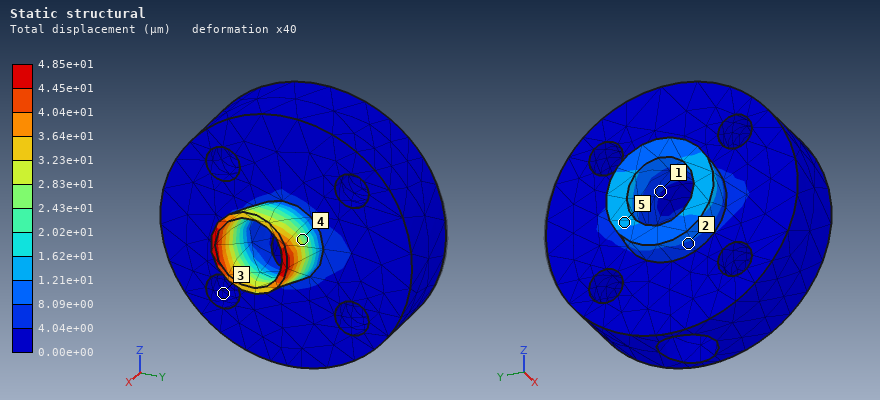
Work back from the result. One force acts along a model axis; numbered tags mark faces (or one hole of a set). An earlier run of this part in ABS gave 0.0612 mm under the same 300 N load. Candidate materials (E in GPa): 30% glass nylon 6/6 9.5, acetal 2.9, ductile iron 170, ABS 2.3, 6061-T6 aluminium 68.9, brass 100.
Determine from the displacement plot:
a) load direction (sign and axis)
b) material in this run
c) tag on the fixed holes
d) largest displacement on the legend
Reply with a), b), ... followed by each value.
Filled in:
a) -Y
b) acetal
c) 3
d) 4.85e+01 µm
